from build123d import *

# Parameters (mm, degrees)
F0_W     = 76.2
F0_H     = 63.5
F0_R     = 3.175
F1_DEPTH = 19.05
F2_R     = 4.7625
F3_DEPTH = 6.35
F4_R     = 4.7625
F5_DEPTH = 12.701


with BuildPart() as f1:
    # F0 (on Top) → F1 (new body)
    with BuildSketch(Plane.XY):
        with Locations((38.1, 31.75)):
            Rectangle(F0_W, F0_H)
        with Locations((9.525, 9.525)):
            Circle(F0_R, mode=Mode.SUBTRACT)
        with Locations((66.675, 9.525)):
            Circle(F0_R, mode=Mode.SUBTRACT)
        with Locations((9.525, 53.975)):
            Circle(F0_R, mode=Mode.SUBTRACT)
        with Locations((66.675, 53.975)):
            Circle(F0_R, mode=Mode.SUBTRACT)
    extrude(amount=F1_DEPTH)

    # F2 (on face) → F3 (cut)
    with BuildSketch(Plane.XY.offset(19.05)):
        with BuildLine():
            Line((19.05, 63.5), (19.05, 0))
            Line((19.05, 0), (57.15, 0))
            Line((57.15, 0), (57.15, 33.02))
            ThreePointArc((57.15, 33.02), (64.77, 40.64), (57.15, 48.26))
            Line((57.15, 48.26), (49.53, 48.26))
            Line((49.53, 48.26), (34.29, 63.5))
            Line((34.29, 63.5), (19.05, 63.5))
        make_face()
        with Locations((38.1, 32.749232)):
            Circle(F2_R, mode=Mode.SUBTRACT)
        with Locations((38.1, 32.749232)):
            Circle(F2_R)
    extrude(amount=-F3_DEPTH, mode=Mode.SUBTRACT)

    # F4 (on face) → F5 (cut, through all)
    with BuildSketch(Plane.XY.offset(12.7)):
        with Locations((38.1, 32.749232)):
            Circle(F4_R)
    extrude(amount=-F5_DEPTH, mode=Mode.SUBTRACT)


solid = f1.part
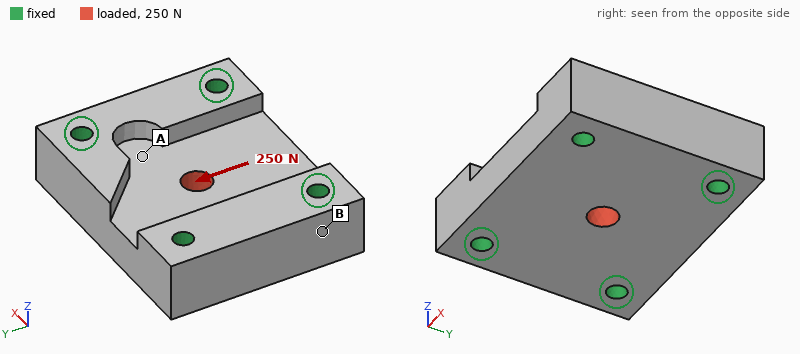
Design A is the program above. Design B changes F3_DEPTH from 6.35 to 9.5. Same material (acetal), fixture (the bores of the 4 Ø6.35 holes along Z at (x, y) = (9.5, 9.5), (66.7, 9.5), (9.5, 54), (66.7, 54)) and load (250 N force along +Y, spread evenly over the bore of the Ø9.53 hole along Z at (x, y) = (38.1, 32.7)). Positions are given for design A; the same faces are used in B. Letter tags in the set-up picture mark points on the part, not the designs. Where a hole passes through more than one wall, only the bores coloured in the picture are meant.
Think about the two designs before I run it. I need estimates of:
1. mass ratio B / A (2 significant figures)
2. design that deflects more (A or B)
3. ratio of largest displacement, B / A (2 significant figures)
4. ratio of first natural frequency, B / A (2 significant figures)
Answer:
0.91
B
1.3
0.97
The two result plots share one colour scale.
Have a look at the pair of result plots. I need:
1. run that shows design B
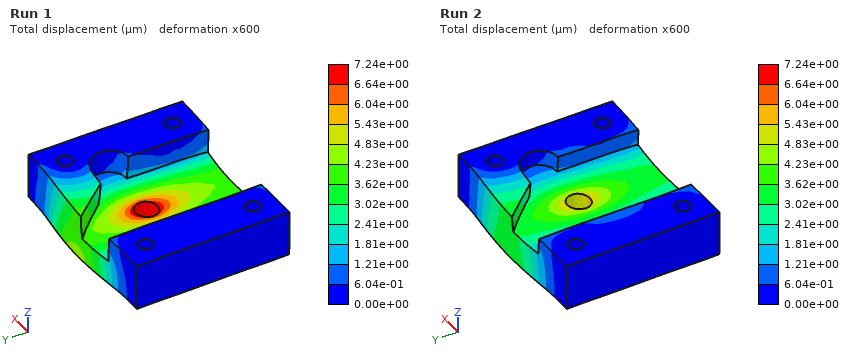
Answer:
Run 1
